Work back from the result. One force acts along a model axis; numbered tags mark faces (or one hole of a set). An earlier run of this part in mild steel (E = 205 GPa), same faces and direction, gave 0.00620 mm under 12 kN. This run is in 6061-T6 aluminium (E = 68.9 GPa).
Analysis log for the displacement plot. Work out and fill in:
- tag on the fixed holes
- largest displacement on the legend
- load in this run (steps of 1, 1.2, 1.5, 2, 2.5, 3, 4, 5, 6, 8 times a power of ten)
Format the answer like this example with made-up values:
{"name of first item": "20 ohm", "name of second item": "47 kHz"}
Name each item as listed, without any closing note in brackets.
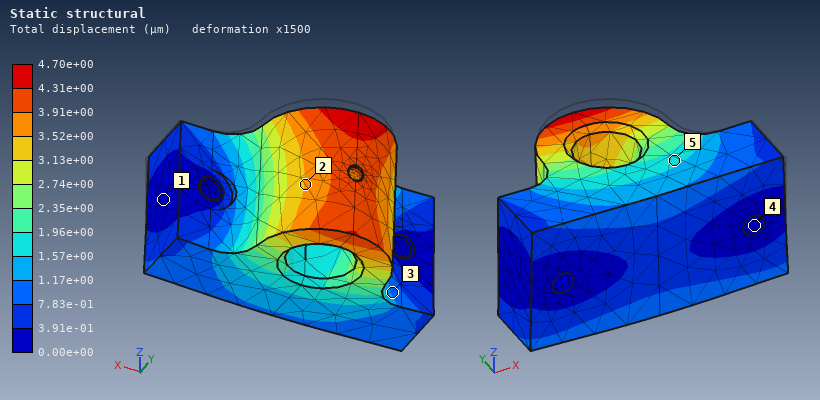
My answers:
{"tag on the fixed holes": "4", "largest displacement on the legend": "4.70e+00 µm", "load in this run": "3 kN"}
